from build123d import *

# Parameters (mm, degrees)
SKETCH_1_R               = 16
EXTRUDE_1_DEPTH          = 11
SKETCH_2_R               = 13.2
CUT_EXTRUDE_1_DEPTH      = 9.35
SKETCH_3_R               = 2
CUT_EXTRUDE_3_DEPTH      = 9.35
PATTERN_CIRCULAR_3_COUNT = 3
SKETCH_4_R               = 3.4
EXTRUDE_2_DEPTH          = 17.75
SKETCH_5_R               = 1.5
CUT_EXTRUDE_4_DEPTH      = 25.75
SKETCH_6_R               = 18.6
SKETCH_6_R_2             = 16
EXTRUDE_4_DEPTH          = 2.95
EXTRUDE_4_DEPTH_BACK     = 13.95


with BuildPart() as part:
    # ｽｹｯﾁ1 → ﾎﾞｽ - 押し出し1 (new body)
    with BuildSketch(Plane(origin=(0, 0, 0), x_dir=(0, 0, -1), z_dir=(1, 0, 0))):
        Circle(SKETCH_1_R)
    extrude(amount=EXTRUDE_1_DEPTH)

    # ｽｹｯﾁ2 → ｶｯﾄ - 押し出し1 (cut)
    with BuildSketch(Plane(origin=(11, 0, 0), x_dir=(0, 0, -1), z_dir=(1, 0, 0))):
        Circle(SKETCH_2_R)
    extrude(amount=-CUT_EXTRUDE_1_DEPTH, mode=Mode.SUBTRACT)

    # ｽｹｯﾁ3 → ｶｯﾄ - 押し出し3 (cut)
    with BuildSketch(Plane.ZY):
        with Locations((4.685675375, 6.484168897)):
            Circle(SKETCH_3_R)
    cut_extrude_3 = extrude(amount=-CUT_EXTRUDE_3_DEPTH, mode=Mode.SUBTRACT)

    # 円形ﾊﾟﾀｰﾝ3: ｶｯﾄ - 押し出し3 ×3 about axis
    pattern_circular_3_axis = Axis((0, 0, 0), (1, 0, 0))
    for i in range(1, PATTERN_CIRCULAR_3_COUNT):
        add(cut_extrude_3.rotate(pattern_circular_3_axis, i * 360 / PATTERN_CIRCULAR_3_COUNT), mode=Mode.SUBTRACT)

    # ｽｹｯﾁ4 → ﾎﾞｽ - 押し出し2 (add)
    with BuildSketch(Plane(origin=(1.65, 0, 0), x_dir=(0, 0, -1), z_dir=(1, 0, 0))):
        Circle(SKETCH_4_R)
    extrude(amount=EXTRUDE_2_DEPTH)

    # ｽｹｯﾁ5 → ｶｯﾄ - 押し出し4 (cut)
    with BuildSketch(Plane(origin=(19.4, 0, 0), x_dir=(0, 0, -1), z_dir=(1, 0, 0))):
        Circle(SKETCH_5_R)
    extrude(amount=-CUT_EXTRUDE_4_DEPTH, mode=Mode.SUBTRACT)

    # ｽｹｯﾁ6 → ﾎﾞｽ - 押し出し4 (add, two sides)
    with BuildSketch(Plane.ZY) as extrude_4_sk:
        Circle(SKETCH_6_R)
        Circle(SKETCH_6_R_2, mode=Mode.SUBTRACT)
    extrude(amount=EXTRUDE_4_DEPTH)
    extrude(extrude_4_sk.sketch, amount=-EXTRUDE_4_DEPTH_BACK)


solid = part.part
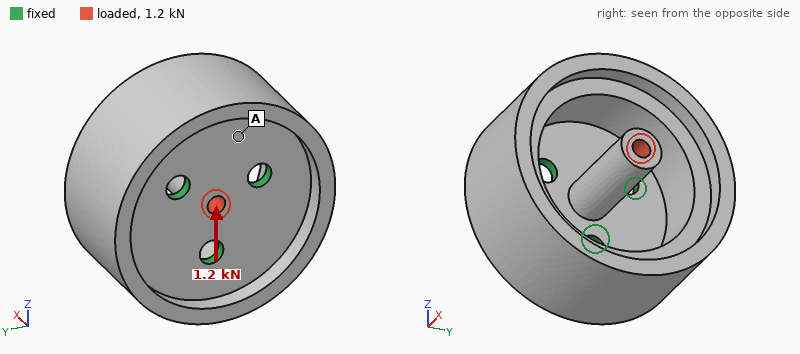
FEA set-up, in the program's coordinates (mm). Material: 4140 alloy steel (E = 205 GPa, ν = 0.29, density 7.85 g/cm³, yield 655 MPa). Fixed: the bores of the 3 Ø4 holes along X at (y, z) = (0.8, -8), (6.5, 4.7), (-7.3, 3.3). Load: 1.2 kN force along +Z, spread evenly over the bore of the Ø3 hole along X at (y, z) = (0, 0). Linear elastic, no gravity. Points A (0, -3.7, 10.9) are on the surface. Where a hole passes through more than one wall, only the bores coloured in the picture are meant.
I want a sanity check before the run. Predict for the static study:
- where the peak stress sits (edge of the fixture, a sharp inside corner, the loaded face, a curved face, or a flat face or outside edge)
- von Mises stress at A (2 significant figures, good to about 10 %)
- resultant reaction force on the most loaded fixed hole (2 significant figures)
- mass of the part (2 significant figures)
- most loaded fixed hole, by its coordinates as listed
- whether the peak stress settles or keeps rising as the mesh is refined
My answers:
edge of the fixture
46 MPa
1.2 kN
70 g
(0.8, -8)
keeps rising
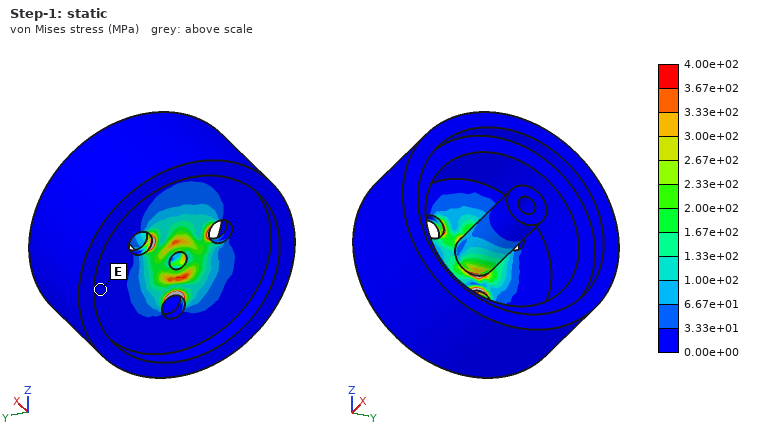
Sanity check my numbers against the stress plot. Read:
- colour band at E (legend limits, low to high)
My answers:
0.00e+00 to 3.33e+01 MPa
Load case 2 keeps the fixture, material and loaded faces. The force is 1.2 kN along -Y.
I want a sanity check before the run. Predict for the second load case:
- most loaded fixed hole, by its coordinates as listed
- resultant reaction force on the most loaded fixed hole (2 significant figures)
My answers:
(-7.3, 3.3)
1.1 kN
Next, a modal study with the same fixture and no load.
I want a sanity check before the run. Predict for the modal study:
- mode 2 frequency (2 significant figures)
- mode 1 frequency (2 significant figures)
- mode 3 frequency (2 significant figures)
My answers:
6100 Hz
6100 Hz
9300 Hz
